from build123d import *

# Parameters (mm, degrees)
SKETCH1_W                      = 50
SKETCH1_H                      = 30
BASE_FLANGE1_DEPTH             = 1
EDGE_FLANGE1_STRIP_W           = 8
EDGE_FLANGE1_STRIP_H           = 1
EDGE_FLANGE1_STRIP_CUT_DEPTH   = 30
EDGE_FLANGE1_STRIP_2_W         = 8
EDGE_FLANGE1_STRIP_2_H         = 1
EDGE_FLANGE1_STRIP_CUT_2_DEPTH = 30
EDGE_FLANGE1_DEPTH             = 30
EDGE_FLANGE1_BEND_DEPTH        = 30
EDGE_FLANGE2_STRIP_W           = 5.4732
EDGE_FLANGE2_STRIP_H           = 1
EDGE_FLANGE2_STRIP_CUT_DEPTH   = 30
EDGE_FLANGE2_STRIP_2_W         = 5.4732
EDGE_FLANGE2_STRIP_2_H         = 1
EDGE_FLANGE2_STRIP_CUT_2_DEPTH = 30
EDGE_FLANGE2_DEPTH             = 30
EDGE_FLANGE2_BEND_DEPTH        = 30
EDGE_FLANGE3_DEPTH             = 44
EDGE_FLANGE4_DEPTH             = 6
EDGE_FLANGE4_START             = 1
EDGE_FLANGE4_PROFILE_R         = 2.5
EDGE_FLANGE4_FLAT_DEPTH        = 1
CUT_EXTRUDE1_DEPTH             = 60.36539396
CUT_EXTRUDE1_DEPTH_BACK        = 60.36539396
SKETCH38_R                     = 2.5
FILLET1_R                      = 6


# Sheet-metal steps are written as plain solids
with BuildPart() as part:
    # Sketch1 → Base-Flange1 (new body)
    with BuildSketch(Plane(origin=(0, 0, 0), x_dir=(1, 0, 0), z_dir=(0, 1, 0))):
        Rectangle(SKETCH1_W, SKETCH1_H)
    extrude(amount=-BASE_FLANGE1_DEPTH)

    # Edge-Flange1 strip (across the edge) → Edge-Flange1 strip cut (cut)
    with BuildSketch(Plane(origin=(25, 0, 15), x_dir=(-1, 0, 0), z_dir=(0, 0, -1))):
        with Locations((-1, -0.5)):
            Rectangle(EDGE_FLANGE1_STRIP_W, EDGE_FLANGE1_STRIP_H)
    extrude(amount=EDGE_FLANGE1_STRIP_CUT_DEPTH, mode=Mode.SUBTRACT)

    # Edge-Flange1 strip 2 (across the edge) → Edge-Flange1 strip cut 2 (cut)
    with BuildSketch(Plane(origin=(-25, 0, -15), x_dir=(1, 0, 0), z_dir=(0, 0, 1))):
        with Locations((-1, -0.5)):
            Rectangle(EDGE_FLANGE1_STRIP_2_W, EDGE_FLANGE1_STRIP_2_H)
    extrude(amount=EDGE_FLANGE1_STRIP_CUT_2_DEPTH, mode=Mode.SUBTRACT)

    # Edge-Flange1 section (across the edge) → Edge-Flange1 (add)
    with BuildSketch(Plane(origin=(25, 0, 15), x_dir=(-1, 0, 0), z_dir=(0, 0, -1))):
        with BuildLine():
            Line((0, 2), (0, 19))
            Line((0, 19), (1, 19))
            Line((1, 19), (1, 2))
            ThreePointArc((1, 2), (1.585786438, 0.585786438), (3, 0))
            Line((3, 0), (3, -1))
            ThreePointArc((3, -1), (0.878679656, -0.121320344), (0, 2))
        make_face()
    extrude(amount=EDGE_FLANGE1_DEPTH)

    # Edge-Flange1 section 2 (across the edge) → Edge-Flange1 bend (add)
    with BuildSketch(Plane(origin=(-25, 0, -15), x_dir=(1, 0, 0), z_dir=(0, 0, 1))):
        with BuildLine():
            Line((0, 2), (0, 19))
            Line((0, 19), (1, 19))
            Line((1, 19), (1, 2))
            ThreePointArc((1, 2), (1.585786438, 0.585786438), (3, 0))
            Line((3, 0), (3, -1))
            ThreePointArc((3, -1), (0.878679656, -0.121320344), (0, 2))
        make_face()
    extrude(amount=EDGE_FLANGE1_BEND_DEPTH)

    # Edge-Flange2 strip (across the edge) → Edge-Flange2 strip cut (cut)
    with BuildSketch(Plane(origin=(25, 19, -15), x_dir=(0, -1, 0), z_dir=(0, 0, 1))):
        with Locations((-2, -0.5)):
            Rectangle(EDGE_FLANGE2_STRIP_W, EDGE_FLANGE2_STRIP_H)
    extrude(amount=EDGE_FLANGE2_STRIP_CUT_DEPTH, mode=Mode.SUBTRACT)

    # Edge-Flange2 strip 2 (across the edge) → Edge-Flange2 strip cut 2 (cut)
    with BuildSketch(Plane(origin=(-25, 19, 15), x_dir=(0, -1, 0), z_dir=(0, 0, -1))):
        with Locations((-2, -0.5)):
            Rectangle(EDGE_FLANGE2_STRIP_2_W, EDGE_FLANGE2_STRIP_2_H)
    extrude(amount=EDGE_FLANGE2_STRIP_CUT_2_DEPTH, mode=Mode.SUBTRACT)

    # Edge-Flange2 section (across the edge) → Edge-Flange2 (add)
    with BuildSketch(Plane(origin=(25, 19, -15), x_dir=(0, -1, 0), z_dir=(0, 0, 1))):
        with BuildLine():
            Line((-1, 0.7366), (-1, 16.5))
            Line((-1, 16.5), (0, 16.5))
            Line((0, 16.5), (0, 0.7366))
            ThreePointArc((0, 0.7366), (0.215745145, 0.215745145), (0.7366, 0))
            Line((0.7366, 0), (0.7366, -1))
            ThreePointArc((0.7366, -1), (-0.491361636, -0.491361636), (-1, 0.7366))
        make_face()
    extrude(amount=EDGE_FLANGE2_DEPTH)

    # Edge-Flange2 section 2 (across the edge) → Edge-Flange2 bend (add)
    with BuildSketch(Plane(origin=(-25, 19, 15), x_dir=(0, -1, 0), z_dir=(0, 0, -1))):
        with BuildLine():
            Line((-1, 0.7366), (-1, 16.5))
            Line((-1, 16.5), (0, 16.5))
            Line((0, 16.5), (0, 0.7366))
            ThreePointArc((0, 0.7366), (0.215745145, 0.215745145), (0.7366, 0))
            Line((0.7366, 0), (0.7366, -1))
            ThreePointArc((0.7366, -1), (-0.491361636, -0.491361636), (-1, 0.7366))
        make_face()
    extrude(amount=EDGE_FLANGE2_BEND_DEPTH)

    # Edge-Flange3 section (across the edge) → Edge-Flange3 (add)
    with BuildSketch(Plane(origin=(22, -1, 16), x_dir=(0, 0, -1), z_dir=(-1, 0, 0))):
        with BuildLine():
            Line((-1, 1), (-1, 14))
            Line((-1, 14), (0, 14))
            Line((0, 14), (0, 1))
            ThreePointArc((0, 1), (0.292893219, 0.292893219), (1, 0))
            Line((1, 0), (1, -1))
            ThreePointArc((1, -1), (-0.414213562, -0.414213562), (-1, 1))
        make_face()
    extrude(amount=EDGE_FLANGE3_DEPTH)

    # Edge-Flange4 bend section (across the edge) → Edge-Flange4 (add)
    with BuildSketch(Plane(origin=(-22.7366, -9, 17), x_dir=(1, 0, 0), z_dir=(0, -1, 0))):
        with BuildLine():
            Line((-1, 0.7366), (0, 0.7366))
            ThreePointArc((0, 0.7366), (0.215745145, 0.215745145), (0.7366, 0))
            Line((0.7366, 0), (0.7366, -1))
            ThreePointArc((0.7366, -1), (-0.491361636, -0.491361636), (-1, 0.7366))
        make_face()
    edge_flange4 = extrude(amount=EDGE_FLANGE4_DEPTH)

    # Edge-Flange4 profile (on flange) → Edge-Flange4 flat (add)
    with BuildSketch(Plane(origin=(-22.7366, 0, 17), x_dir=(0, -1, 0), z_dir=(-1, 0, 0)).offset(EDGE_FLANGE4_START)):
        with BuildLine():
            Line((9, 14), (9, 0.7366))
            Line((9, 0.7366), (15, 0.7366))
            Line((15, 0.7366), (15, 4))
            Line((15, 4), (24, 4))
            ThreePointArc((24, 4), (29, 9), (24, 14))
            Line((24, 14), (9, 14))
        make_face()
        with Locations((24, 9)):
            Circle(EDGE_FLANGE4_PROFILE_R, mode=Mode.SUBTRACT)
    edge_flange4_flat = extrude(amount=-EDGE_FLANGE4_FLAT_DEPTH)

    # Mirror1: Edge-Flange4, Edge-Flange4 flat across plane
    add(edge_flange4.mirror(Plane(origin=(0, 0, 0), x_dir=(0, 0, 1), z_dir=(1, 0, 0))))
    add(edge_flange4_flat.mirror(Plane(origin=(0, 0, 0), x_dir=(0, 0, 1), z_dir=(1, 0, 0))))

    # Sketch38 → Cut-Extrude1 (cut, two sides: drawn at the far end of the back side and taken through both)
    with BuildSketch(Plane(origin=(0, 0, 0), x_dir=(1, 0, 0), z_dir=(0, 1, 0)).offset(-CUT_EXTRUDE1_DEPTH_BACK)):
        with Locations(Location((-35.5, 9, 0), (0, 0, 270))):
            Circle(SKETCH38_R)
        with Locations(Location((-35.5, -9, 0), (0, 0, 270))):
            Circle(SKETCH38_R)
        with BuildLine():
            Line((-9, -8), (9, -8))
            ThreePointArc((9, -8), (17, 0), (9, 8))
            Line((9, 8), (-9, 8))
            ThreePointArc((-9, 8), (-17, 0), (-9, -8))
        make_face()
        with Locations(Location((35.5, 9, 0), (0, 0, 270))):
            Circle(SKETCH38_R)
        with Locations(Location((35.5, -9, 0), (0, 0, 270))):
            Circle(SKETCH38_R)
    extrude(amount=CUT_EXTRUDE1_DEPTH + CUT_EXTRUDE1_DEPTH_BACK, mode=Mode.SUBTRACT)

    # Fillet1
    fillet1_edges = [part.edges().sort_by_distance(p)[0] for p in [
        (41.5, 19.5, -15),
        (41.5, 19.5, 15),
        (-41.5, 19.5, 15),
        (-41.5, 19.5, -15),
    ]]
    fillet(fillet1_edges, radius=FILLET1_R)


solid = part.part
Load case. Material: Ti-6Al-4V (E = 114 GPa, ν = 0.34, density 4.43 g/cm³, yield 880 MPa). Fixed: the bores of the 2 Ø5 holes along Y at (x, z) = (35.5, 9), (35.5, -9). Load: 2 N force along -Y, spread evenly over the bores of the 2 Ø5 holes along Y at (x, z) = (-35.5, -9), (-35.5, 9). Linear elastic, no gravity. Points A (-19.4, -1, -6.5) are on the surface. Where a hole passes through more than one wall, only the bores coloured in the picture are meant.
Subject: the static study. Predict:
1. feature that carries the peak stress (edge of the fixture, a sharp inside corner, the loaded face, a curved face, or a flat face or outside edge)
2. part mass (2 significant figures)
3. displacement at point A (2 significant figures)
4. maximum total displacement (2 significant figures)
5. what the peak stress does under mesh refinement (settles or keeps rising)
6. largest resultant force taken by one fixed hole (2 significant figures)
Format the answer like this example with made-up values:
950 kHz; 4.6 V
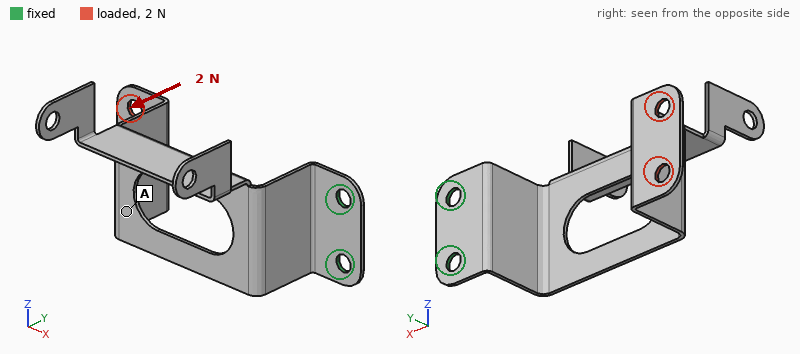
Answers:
a sharp inside corner; 18 g; 0.73 mm; 1.2 mm; keeps rising; 1.6 N
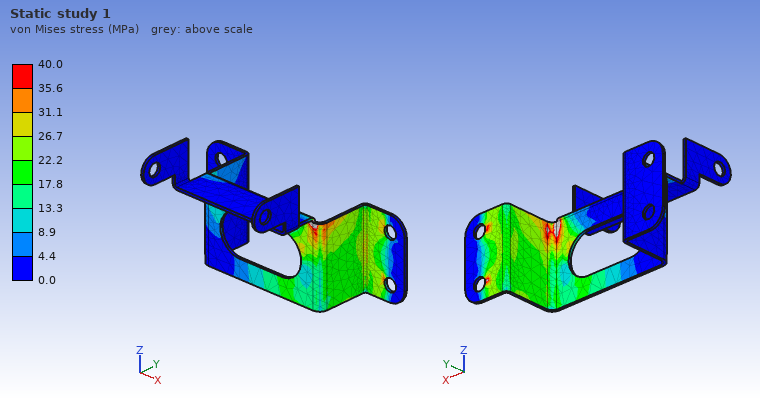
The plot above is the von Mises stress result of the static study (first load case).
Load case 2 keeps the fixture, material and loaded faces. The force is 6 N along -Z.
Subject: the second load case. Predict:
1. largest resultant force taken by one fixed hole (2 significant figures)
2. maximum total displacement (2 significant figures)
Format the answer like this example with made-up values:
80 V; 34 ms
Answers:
20 N; 1.2 mm
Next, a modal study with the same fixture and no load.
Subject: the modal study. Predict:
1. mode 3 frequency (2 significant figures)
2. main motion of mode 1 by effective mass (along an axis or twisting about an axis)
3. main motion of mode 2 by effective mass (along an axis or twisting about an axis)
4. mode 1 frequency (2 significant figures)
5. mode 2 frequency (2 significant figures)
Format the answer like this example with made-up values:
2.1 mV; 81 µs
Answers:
350 Hz; along Y; along Z; 88 Hz; 180 Hz
